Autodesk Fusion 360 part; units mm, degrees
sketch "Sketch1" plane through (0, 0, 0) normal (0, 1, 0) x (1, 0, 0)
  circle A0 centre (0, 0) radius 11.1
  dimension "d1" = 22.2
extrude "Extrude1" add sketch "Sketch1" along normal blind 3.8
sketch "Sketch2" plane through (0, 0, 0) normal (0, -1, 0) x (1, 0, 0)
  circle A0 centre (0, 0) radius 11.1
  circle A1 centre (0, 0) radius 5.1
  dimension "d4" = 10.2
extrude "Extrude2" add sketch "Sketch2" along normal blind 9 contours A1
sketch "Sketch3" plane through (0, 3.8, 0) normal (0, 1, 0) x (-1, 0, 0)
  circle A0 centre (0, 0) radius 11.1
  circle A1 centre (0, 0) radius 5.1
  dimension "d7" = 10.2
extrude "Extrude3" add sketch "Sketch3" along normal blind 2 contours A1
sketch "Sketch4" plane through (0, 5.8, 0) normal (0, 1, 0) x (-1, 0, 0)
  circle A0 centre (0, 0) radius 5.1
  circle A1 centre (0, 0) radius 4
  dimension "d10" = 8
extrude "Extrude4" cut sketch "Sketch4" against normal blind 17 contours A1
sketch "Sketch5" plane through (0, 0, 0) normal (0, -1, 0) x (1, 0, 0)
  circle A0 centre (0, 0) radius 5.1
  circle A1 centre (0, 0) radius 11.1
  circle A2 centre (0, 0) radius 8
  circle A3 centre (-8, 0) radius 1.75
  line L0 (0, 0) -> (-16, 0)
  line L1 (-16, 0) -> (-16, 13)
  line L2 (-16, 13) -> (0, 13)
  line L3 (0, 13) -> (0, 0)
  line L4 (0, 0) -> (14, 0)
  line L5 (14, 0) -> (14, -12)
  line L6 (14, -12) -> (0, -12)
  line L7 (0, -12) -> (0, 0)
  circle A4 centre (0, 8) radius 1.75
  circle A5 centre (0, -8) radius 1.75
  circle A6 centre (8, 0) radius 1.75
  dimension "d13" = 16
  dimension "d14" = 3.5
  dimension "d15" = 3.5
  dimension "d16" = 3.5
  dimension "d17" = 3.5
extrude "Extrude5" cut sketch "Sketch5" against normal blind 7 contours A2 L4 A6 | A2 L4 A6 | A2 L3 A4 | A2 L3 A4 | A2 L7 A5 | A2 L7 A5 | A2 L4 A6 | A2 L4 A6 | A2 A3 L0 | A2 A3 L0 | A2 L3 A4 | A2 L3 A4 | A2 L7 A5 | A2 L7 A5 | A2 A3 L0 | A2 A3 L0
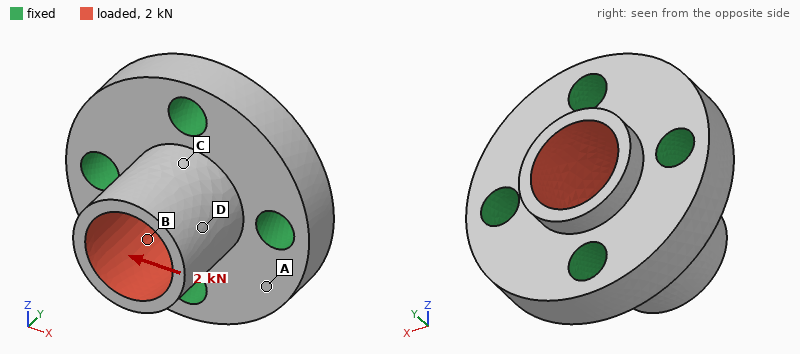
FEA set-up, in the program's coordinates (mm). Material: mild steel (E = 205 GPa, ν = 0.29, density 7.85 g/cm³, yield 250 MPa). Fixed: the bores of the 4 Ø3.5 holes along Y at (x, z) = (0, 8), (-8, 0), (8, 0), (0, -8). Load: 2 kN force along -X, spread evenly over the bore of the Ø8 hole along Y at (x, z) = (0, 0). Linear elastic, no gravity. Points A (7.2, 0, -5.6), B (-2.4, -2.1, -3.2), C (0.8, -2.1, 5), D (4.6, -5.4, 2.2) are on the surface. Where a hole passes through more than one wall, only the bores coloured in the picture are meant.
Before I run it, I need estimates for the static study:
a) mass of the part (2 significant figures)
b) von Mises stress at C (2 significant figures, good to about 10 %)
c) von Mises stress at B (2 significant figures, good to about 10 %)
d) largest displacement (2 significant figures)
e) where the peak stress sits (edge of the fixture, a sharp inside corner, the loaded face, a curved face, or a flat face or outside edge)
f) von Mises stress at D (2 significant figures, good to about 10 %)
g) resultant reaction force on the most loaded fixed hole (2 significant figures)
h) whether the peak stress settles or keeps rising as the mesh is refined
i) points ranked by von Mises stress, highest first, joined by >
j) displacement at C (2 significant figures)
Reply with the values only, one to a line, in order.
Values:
12 g
73 MPa
100 MPa
8.9 µm
a sharp inside corner
31 MPa
750 N
keeps rising
B > C > D > A
2.8 µm
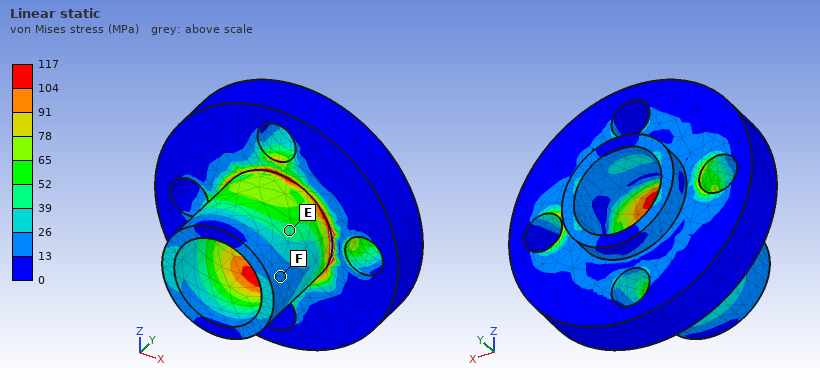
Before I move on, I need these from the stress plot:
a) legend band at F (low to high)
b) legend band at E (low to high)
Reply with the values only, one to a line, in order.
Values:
13 to 26 MPa
39 to 52 MPa
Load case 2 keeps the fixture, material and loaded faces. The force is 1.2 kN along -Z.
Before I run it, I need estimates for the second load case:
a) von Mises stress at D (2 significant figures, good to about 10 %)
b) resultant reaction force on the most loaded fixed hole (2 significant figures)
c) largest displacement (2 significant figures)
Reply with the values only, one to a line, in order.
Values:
28 MPa
450 N
5.4 µm
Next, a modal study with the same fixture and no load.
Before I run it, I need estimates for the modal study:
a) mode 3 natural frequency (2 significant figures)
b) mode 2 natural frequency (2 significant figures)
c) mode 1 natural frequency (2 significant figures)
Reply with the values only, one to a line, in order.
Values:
46 kHz
46 kHz
45 kHz
